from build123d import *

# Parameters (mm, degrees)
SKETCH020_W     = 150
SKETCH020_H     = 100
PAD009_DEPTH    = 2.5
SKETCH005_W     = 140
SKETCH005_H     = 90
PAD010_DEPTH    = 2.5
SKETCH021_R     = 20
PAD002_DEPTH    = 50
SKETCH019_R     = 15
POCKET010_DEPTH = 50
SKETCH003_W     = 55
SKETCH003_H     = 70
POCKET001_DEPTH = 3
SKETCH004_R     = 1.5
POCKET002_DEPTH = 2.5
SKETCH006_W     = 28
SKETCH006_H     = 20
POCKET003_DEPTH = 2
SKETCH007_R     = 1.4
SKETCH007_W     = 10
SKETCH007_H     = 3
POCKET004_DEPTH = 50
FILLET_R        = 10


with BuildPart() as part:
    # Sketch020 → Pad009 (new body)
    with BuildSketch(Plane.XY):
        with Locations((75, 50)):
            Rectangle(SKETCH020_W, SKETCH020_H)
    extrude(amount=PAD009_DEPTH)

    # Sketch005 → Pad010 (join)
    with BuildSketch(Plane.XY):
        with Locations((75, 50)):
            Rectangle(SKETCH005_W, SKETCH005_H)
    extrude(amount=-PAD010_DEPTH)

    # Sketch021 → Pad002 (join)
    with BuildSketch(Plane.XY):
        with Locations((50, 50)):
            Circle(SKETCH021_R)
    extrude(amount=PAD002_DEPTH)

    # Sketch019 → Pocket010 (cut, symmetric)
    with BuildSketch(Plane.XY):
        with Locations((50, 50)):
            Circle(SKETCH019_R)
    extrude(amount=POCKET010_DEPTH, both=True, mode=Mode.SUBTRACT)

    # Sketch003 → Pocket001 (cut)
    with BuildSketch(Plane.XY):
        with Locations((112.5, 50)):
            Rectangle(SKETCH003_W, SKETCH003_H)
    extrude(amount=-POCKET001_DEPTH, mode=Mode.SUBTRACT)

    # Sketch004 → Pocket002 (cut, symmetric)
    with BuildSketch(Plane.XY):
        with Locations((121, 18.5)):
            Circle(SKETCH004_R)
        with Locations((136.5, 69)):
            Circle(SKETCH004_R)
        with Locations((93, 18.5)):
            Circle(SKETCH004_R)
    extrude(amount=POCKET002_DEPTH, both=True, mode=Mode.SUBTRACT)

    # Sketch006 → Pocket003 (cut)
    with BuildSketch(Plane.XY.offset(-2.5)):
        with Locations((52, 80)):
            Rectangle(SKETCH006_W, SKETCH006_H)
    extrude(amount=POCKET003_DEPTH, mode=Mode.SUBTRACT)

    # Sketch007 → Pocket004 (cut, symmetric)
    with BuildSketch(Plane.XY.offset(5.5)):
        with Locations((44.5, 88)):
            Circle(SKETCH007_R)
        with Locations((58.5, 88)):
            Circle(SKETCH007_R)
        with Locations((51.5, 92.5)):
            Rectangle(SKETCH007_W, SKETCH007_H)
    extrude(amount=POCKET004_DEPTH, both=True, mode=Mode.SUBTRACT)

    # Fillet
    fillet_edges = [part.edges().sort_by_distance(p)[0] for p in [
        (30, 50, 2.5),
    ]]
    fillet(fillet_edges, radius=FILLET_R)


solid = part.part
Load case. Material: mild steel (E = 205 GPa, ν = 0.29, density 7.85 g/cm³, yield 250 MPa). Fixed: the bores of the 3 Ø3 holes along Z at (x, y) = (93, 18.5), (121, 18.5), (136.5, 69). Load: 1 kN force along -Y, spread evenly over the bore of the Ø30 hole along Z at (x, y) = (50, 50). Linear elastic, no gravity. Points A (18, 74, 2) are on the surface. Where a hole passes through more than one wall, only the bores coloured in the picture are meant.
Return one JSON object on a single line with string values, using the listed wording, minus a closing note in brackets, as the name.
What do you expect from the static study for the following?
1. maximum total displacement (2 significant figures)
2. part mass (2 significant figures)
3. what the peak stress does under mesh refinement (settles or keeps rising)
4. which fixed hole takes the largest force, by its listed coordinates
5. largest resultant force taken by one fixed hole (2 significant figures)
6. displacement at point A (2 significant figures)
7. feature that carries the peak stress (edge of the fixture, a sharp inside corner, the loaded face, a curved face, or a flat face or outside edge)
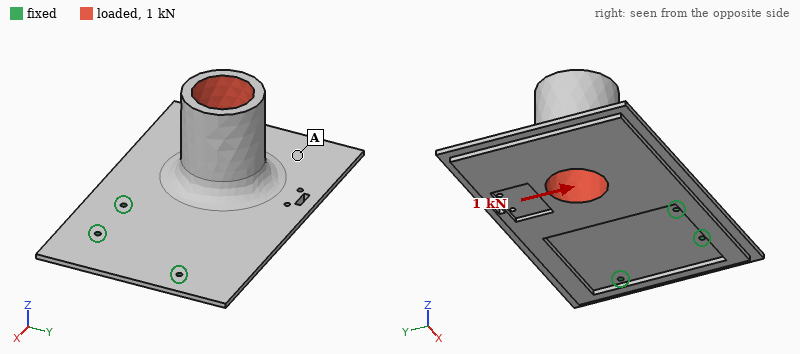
{"maximum total displacement": "0.79 mm", "part mass": "660 g", "what the peak stress does under mesh refinement": "keeps rising", "which fixed hole takes the largest force, by its listed coordinates": "(93, 18.5)", "largest resultant force taken by one fixed hole": "1.1 kN", "displacement at point A": "0.55 mm", "feature that carries the peak stress": "edge of the fixture"}
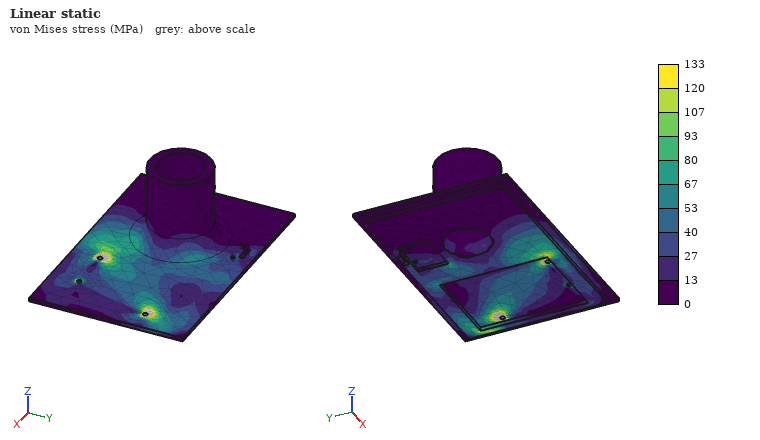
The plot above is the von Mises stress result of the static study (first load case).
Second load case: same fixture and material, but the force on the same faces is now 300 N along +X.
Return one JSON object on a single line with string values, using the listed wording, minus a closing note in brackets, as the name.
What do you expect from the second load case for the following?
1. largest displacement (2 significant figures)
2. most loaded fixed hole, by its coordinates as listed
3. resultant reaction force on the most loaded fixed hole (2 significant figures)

{"largest displacement": "0.32 mm", "most loaded fixed hole, by its coordinates as listed": "(93, 18.5)", "resultant reaction force on the most loaded fixed hole": "310 N"}
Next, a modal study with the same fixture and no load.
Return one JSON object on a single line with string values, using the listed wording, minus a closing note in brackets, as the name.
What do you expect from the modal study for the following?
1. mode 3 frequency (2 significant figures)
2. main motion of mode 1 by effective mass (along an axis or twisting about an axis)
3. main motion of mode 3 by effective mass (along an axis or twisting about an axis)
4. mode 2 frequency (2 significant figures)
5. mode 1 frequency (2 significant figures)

{"mode 3 frequency": "1600 Hz", "main motion of mode 1 by effective mass": "along Z", "main motion of mode 3 by effective mass": "along Z", "mode 2 frequency": "540 Hz", "mode 1 frequency": "180 Hz"}
